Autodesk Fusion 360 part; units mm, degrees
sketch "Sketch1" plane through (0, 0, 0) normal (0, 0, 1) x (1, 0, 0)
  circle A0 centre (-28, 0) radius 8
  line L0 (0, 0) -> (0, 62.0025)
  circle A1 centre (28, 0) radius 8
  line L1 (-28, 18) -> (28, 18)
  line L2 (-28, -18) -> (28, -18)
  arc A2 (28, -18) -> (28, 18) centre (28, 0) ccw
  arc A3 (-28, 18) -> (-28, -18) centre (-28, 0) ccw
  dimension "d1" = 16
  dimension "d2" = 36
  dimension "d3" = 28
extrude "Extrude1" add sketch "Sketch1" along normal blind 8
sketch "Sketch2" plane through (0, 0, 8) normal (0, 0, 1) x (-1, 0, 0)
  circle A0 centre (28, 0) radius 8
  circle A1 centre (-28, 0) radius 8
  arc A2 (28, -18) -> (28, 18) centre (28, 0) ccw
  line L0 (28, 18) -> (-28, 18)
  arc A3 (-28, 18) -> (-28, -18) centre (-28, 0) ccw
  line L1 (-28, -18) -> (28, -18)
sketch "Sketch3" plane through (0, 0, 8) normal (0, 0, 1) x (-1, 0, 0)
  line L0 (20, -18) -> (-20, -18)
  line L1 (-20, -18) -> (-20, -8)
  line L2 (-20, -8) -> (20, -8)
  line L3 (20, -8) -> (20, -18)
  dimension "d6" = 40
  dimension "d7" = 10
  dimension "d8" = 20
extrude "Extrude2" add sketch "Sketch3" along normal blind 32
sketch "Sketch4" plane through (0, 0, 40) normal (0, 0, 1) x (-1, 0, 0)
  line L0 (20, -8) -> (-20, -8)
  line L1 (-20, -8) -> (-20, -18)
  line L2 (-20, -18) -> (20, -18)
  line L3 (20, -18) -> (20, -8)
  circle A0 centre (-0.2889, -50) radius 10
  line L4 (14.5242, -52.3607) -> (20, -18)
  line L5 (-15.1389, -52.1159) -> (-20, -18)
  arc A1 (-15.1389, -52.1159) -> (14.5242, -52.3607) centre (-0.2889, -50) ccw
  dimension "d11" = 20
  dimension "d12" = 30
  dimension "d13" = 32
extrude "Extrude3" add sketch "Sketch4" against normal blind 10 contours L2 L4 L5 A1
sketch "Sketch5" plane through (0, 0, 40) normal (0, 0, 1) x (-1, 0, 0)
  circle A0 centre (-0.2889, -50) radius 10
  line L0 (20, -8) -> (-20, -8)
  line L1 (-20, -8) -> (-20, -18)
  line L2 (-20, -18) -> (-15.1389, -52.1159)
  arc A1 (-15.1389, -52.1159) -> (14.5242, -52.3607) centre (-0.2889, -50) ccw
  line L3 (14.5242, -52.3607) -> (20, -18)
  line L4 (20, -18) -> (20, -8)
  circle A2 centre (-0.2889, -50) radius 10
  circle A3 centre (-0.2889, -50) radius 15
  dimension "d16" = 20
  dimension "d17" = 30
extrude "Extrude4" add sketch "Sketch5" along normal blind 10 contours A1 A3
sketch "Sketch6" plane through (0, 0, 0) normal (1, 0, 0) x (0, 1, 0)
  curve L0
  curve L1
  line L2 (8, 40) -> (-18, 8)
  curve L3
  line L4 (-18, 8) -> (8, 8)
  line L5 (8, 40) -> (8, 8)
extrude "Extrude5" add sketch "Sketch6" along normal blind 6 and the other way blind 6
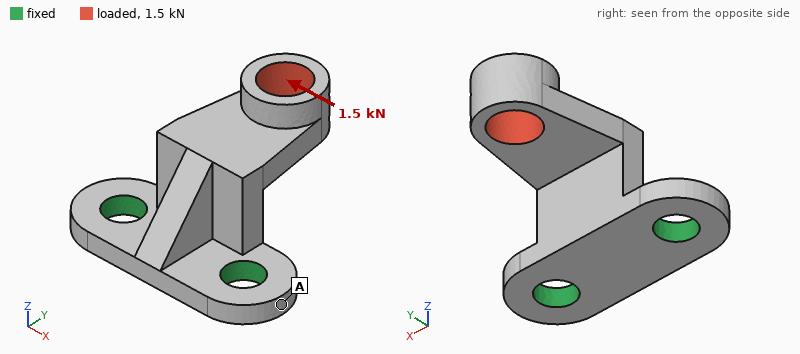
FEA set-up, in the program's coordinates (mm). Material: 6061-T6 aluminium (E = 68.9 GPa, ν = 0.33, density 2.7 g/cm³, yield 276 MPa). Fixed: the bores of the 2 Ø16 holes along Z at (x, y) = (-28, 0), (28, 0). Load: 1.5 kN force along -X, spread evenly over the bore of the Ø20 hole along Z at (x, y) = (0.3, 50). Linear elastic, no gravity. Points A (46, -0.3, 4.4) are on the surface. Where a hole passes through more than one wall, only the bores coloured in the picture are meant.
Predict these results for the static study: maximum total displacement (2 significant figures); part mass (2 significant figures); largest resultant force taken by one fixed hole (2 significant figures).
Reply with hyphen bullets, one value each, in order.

- 0.16 mm
- 150 g
- 2.0 kN
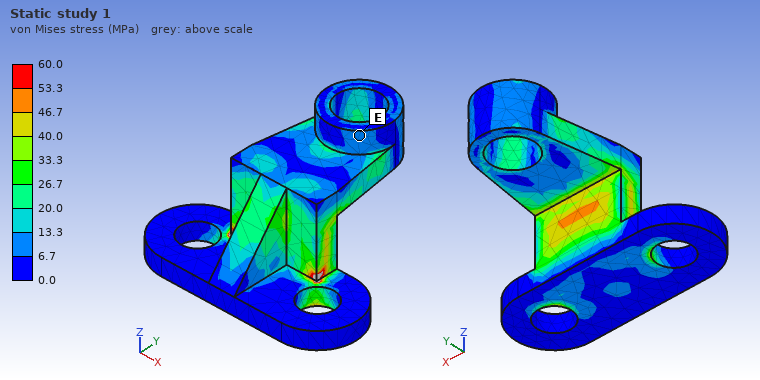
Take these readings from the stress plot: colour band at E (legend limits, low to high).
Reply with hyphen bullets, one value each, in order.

- 6.7 to 13.3 MPa
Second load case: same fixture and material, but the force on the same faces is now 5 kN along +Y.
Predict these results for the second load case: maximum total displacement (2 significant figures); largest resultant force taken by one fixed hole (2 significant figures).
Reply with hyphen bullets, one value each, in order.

- 0.66 mm
- 2.6 kN
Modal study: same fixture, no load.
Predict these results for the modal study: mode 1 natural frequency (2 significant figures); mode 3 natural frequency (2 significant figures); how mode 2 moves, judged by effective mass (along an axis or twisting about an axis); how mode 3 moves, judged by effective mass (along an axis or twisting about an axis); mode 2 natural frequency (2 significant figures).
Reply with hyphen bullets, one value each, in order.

- 2000 Hz
- 5100 Hz
- along X
- along Y
- 3300 Hz
